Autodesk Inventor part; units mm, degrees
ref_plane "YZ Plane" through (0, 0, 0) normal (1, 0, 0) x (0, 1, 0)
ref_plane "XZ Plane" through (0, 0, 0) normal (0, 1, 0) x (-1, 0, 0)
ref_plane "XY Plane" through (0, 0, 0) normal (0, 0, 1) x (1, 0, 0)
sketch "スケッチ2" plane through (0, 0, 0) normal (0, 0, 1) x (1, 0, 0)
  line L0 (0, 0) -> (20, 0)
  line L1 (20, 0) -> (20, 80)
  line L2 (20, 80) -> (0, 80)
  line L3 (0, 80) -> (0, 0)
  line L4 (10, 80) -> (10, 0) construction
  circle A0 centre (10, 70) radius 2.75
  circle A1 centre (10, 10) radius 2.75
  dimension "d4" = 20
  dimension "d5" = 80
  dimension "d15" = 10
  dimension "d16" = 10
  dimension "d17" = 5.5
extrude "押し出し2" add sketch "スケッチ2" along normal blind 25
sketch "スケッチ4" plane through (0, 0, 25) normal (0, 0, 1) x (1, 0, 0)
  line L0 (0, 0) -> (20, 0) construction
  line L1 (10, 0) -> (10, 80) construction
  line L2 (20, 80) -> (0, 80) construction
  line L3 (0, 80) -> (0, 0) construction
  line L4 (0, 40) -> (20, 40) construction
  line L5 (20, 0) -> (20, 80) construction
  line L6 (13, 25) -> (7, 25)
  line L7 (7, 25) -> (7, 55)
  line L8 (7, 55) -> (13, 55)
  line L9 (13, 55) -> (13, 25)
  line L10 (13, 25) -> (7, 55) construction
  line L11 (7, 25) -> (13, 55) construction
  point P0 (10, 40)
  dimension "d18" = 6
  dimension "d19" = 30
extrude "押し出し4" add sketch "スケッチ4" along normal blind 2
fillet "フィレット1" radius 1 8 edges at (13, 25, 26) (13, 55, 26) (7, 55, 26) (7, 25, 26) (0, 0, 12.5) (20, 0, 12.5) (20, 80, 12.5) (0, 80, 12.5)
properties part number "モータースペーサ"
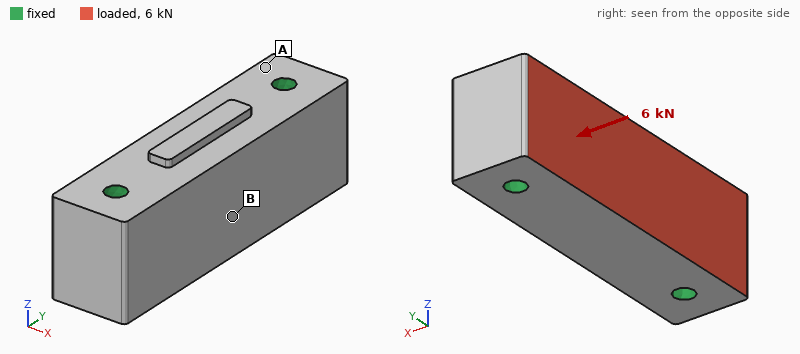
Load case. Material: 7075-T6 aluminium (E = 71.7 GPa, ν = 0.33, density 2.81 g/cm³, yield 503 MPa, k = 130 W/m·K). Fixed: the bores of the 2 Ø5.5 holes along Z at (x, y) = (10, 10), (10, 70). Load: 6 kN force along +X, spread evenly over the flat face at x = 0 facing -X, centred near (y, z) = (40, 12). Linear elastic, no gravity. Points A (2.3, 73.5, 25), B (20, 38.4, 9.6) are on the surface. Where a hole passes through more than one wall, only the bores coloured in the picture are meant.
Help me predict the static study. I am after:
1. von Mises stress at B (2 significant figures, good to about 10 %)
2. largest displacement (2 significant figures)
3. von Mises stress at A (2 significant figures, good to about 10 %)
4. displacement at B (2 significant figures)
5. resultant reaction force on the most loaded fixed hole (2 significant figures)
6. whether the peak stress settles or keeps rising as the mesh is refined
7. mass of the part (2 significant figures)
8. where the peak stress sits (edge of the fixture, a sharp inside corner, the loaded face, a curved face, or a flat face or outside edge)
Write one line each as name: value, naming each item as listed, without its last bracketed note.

von Mises stress at B: 11 MPa
largest displacement: 7.4 µm
von Mises stress at A: 4.9 MPa
displacement at B: 6.5 µm
resultant reaction force on the most loaded fixed hole: 3.0 kN
whether the peak stress settles or keeps rising as the mesh is refined: keeps rising
mass of the part: 110 g
where the peak stress sits: edge of the fixture
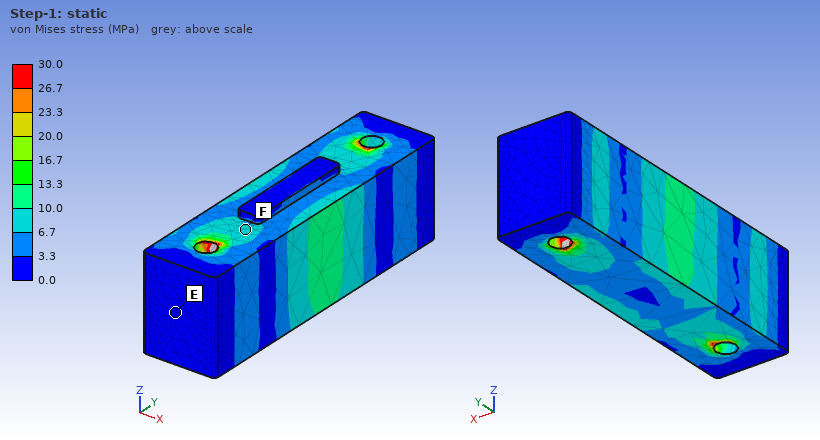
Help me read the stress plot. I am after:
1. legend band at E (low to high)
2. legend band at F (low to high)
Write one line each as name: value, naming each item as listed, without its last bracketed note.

legend band at E: 0.0 to 3.3 MPa
legend band at F: 6.7 to 10.0 MPa
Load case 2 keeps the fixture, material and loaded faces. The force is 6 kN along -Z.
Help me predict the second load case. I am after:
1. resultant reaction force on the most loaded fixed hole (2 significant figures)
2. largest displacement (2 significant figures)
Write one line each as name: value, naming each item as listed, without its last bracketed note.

resultant reaction force on the most loaded fixed hole: 3.0 kN
largest displacement: 11 µm
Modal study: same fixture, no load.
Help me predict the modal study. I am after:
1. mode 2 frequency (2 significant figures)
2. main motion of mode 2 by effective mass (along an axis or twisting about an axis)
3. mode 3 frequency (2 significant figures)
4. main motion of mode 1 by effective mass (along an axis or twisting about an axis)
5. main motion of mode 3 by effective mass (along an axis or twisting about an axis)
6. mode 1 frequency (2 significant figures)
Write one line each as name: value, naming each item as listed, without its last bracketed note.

mode 2 frequency: 20 kHz
main motion of mode 2 by effective mass: along Z
mode 3 frequency: 23 kHz
main motion of mode 1 by effective mass: along X
main motion of mode 3 by effective mass: twisting about Y
mode 1 frequency: 15 kHz
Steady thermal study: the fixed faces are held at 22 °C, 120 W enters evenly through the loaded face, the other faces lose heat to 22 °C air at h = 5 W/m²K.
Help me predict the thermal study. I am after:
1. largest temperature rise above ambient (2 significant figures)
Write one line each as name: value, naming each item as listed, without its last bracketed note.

largest temperature rise above ambient: 14 K
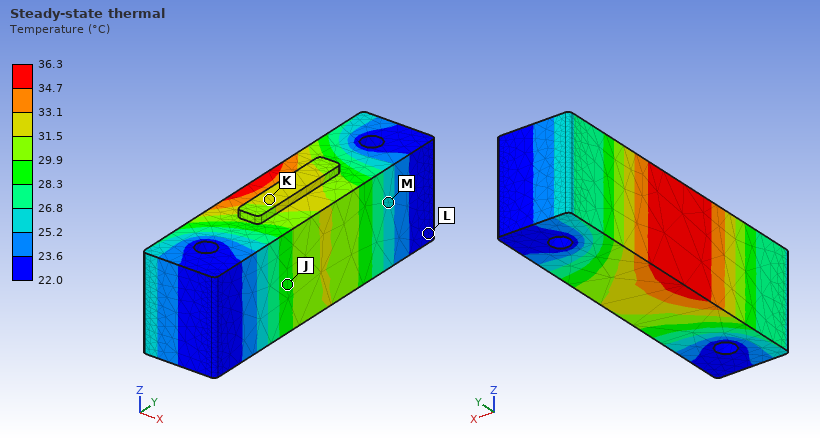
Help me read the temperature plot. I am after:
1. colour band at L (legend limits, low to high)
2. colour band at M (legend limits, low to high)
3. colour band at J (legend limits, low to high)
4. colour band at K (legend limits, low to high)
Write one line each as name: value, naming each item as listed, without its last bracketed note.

colour band at L: 22.0 to 23.6 °C
colour band at M: 25.2 to 26.8 °C
colour band at J: 28.3 to 29.9 °C
colour band at K: 31.5 to 33.1 °C
